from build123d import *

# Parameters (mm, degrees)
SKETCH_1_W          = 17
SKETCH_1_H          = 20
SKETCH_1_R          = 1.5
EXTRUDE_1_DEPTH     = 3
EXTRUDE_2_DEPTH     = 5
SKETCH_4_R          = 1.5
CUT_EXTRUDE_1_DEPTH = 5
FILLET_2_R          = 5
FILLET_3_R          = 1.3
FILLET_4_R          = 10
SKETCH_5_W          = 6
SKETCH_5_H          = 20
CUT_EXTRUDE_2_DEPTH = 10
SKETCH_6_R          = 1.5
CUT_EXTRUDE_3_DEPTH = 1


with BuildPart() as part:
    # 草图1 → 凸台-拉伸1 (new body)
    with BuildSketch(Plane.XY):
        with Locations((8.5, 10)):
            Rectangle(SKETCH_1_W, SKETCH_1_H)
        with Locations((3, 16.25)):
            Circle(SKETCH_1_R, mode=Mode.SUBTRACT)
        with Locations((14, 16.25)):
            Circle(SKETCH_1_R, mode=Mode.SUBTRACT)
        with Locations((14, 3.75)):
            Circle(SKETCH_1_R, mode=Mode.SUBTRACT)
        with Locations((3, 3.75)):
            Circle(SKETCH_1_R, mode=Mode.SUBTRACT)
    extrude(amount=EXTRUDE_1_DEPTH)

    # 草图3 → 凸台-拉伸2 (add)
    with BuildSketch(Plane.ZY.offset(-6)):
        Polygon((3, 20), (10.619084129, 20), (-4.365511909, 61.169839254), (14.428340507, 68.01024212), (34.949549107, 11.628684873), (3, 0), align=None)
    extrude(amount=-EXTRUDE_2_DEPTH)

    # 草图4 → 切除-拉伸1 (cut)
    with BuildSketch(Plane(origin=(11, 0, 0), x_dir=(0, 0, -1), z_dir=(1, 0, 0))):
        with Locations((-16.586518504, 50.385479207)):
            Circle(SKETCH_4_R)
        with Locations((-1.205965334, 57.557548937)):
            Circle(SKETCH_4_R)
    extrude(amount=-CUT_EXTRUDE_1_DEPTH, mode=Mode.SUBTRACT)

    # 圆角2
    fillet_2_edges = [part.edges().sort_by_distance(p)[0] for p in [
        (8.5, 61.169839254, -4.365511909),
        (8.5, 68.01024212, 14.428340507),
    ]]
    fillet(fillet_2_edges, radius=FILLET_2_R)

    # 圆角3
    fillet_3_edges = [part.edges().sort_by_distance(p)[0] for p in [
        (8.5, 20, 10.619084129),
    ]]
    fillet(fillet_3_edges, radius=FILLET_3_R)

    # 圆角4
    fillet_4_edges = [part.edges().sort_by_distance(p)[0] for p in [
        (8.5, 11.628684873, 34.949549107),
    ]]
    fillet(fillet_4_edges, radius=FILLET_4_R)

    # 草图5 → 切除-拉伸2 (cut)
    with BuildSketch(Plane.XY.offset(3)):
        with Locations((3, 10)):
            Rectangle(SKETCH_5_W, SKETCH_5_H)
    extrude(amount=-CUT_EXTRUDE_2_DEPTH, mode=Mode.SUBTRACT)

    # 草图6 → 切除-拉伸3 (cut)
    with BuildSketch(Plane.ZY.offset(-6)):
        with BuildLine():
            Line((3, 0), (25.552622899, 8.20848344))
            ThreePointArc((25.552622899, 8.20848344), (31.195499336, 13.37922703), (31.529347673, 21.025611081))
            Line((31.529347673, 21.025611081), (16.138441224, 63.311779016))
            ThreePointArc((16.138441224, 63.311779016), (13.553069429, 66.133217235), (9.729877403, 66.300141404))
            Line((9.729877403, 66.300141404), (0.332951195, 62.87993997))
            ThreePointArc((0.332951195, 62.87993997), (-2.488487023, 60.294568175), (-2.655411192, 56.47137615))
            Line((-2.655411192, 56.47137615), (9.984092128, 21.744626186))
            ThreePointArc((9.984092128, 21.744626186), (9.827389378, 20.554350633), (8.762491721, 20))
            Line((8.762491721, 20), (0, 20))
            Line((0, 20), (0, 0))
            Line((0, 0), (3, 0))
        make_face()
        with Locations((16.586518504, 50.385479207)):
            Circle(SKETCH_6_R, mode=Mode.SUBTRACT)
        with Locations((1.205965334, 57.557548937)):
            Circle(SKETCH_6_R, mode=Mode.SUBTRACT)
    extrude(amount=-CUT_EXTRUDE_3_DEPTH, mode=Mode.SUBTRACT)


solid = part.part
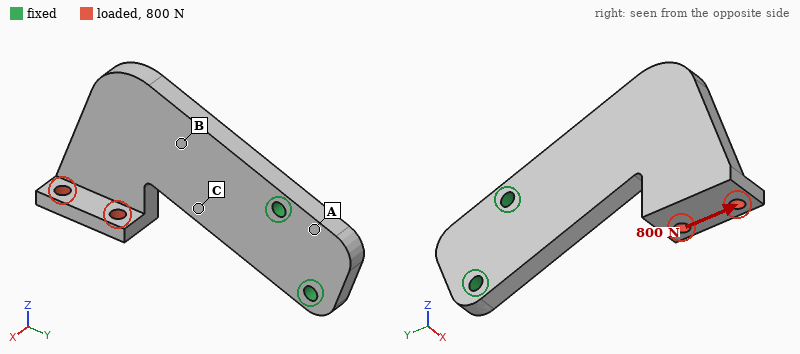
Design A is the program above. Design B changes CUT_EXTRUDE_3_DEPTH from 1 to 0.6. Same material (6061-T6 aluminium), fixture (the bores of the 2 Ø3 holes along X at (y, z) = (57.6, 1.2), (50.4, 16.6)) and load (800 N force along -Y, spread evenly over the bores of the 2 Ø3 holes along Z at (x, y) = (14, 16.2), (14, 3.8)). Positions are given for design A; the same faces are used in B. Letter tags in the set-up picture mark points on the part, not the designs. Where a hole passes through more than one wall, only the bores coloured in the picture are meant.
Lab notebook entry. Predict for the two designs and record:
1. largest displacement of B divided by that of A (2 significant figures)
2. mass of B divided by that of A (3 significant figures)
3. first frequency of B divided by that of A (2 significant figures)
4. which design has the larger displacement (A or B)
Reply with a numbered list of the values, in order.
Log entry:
1. 0.80
2. 1.09
3. 1.1
4. A
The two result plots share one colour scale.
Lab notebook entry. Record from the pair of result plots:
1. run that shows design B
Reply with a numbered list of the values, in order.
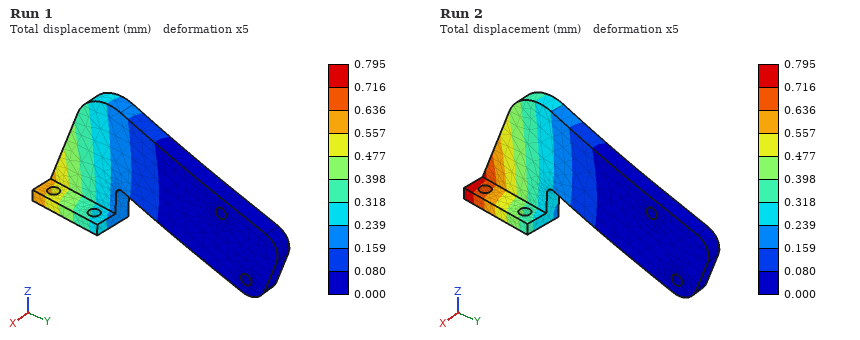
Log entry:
1. Run 1
